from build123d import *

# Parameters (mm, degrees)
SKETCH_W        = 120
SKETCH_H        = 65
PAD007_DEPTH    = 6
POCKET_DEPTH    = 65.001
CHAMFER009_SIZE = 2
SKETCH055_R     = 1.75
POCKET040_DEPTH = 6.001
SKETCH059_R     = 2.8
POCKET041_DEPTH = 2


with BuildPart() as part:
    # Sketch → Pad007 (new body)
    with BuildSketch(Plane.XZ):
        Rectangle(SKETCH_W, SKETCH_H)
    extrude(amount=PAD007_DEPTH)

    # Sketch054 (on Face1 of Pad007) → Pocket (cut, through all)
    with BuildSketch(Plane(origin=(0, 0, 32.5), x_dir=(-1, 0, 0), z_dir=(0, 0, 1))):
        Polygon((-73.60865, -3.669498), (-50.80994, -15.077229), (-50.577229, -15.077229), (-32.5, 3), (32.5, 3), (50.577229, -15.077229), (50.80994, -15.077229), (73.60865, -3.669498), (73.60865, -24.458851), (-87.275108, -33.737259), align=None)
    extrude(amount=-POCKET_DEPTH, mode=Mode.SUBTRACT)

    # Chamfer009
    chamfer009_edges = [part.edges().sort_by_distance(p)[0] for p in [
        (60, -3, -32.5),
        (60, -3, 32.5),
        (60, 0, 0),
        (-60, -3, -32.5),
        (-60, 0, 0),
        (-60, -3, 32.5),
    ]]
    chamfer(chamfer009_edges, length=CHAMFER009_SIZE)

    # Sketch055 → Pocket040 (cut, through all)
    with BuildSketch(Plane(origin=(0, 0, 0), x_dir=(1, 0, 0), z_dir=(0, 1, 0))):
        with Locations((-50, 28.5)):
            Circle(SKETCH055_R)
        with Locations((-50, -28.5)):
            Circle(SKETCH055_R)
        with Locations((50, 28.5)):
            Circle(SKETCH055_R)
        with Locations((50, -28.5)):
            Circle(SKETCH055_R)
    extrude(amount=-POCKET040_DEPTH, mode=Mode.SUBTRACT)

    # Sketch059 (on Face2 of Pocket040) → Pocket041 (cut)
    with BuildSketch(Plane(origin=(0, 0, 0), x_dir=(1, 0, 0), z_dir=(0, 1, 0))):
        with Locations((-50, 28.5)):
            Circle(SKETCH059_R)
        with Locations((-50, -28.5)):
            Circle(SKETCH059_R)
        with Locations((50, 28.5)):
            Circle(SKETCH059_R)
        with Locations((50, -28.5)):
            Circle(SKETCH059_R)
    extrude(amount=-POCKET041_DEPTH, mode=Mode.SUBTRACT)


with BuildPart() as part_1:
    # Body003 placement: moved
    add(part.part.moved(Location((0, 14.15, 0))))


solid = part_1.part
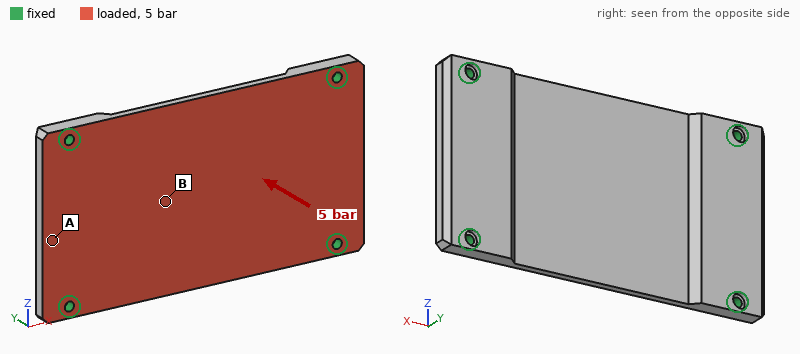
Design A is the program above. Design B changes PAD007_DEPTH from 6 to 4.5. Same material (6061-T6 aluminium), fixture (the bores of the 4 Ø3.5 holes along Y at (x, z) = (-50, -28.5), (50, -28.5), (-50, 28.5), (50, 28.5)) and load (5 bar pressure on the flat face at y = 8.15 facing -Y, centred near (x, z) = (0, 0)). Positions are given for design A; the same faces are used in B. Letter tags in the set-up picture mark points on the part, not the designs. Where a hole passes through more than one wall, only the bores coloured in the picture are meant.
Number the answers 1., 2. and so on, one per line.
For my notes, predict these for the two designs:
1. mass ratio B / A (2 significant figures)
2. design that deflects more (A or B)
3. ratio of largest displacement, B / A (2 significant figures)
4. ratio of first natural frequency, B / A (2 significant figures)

1. 0.65
2. B
3. 4.4
4. 0.70
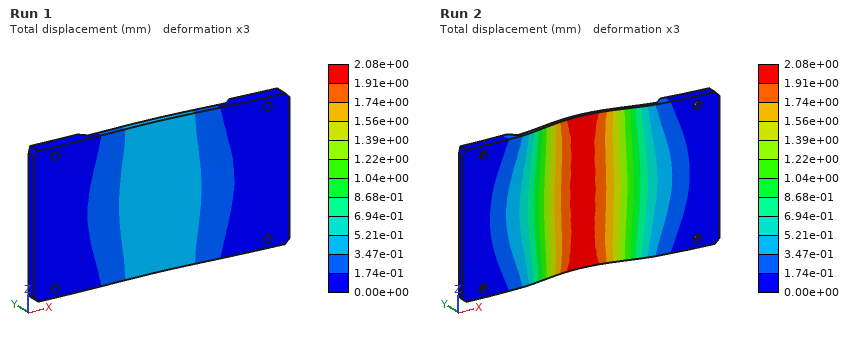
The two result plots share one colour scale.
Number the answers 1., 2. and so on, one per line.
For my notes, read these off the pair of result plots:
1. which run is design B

1. Run 2
